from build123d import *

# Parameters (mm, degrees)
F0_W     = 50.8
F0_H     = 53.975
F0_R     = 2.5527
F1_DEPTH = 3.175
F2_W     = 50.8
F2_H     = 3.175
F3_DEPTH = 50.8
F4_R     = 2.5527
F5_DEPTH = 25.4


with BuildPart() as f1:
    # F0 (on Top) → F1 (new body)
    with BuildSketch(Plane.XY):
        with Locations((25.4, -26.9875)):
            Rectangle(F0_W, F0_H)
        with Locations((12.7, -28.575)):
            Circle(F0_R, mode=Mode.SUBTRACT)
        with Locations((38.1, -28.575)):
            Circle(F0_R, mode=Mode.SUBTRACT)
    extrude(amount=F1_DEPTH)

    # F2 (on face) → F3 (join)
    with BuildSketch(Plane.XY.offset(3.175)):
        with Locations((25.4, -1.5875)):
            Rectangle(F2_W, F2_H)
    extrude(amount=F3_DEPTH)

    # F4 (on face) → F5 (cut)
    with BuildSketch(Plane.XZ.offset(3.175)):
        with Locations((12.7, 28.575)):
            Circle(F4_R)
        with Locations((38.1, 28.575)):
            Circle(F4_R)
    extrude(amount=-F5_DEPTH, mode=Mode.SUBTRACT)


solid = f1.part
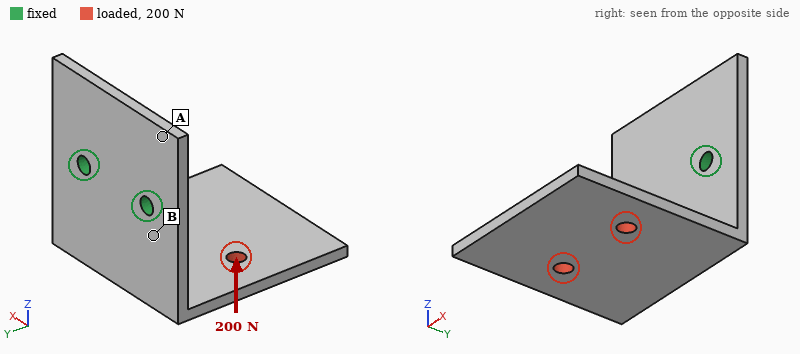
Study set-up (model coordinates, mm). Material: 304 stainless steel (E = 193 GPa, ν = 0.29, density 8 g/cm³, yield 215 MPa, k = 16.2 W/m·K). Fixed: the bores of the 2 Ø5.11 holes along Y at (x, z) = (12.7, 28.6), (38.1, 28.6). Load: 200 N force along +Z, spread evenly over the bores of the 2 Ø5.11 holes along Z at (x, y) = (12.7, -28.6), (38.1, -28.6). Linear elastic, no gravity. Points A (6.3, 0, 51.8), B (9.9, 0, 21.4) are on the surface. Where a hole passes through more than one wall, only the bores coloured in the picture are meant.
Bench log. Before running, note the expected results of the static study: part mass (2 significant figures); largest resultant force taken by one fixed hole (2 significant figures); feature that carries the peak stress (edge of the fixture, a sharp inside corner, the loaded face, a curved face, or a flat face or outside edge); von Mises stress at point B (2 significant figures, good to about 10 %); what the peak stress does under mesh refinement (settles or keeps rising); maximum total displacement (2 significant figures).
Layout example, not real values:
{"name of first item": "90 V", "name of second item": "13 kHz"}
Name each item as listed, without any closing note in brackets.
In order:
{"part mass": "130 g", "largest resultant force taken by one fixed hole": "100 N", "feature that carries the peak stress": "edge of the fixture", "von Mises stress at point B": "60 MPa", "what the peak stress does under mesh refinement": "keeps rising", "maximum total displacement": "0.38 mm"}
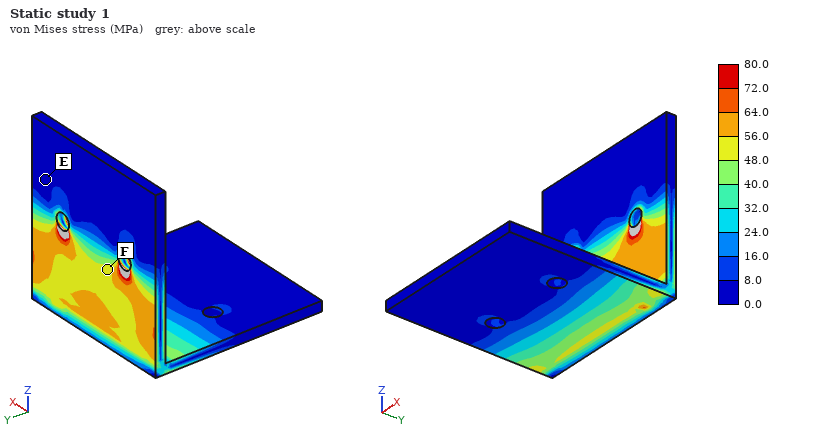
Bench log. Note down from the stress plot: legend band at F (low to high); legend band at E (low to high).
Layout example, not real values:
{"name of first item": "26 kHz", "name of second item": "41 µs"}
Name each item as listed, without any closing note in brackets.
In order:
{"legend band at F": "48.0 to 56.0 MPa", "legend band at E": "0.0 to 8.0 MPa"}
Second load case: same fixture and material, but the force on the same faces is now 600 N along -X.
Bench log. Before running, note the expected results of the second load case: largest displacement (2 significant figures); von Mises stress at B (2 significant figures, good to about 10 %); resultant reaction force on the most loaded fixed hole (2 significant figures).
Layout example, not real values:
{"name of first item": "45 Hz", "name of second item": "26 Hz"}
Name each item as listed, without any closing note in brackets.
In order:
{"largest displacement": "0.30 mm", "von Mises stress at B": "100 MPa", "resultant reaction force on the most loaded fixed hole": "800 N"}
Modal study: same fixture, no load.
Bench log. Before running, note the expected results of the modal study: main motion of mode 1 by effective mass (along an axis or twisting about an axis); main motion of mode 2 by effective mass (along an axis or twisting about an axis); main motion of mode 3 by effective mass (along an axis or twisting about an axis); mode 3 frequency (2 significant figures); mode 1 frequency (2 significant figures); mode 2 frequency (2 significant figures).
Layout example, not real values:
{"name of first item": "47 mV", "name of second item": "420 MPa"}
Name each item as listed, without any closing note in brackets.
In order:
{"main motion of mode 1 by effective mass": "along Z", "main motion of mode 2 by effective mass": "along X", "main motion of mode 3 by effective mass": "along Y", "mode 3 frequency": "1800 Hz", "mode 1 frequency": "520 Hz", "mode 2 frequency": "1000 Hz"}
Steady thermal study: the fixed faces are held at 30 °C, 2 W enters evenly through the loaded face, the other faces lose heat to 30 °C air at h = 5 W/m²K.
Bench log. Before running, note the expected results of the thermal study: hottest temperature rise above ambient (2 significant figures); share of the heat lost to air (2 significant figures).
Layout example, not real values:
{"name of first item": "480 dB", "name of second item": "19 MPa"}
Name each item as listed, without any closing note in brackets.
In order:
{"hottest temperature rise above ambient": "31 K", "share of the heat lost to air": "40 %"}
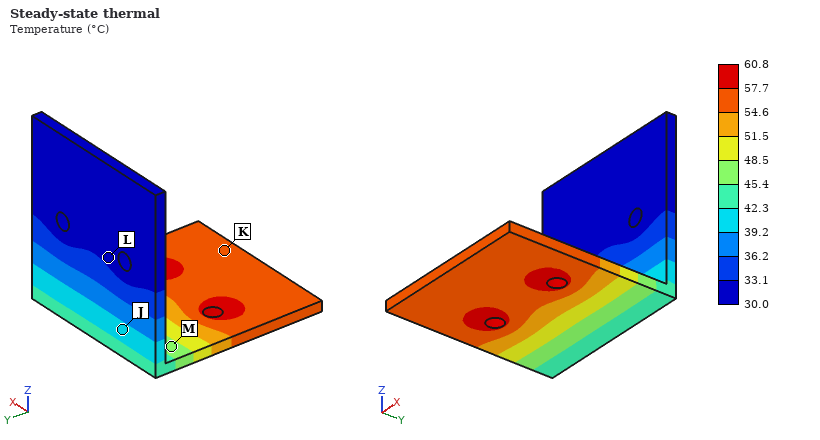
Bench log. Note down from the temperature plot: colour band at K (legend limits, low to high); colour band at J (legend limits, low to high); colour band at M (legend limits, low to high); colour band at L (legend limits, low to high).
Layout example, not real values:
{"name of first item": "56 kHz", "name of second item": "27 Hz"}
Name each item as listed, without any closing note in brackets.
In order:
{"colour band at K": "54.6 to 57.7 °C", "colour band at J": "39.2 to 42.3 °C", "colour band at M": "45.4 to 48.5 °C", "colour band at L": "30.0 to 33.1 °C"}
